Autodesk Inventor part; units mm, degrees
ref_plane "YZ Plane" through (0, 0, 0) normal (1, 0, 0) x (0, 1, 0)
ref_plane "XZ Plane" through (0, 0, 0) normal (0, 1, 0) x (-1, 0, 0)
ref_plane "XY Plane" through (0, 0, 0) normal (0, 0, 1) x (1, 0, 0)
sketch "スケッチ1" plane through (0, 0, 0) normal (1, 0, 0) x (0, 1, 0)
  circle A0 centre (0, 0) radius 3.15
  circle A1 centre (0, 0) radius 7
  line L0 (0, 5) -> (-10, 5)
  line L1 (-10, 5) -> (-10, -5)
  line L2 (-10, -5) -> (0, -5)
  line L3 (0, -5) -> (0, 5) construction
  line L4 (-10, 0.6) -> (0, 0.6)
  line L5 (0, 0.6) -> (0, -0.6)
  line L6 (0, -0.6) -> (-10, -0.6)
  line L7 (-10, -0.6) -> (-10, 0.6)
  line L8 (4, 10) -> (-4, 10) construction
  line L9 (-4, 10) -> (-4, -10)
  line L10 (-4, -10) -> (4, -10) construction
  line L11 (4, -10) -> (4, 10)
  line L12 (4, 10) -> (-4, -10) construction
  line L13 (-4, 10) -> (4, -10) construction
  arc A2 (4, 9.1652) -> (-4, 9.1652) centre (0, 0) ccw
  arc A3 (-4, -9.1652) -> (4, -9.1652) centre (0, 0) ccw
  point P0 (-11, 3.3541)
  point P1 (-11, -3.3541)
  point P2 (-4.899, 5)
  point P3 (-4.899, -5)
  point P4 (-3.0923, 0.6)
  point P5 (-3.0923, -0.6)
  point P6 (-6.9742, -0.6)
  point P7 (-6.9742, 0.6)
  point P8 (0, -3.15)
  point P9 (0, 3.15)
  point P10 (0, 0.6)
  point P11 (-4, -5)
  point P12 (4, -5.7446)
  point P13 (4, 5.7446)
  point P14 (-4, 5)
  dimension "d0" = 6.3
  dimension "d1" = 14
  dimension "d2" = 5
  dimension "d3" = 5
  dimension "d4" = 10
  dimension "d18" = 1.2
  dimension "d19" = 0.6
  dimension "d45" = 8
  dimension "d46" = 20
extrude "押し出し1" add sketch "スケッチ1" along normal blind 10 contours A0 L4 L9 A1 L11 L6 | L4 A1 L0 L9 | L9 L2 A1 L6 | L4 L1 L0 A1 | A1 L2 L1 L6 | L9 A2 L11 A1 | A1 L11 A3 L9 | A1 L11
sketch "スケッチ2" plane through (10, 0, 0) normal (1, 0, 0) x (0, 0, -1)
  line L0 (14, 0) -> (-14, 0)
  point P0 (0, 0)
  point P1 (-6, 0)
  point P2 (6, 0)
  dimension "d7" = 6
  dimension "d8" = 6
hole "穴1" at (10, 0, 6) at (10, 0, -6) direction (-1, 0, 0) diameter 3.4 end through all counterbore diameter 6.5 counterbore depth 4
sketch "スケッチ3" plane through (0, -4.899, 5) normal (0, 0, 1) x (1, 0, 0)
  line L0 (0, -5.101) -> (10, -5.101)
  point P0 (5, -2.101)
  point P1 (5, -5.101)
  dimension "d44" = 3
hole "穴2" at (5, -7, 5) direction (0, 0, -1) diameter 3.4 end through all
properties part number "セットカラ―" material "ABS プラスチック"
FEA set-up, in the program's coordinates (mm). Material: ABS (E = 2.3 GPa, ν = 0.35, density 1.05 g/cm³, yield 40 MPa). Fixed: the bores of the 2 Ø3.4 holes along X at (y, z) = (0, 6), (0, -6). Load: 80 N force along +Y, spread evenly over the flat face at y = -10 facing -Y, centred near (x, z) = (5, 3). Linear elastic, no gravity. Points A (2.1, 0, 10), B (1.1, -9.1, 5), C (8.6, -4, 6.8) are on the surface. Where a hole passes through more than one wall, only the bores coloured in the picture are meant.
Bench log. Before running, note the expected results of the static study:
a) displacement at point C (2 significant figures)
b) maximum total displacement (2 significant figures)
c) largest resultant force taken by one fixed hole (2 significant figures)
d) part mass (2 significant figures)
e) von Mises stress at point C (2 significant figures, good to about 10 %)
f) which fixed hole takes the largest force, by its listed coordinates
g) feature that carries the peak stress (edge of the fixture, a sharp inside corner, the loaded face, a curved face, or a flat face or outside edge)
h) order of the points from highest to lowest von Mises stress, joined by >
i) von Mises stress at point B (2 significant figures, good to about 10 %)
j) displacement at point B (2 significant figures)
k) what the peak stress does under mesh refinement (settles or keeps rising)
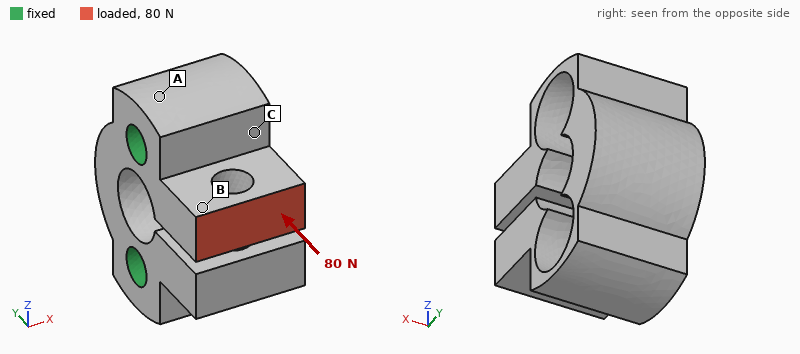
0.020 mm
0.10 mm
78 N
1.6 g
4.2 MPa
(0, 6)
a sharp inside corner
C > B > A
2.5 MPa
0.053 mm
keeps rising
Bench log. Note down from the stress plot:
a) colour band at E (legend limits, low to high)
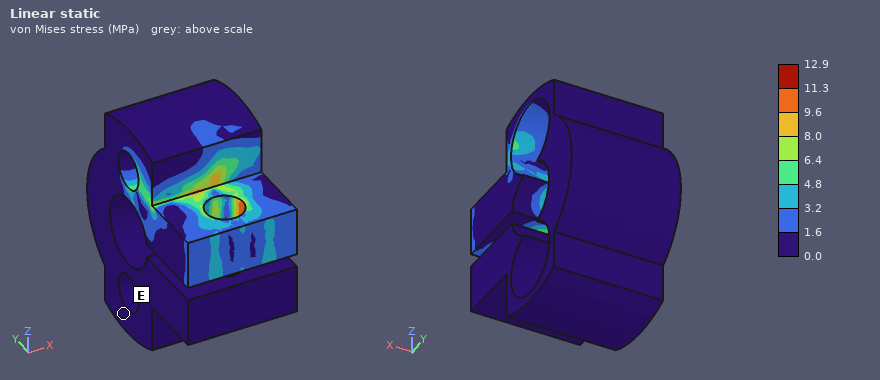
0.0 to 1.6 MPa
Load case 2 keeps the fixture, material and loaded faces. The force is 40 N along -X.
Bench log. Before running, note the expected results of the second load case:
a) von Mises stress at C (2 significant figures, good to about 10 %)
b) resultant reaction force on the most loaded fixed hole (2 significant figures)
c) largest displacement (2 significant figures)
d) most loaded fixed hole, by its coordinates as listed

5.9 MPa
40 N
0.12 mm
(0, 6)
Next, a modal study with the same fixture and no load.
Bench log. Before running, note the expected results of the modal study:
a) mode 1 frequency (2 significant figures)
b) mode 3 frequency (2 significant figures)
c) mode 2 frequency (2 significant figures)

7300 Hz
8700 Hz
7300 Hz
